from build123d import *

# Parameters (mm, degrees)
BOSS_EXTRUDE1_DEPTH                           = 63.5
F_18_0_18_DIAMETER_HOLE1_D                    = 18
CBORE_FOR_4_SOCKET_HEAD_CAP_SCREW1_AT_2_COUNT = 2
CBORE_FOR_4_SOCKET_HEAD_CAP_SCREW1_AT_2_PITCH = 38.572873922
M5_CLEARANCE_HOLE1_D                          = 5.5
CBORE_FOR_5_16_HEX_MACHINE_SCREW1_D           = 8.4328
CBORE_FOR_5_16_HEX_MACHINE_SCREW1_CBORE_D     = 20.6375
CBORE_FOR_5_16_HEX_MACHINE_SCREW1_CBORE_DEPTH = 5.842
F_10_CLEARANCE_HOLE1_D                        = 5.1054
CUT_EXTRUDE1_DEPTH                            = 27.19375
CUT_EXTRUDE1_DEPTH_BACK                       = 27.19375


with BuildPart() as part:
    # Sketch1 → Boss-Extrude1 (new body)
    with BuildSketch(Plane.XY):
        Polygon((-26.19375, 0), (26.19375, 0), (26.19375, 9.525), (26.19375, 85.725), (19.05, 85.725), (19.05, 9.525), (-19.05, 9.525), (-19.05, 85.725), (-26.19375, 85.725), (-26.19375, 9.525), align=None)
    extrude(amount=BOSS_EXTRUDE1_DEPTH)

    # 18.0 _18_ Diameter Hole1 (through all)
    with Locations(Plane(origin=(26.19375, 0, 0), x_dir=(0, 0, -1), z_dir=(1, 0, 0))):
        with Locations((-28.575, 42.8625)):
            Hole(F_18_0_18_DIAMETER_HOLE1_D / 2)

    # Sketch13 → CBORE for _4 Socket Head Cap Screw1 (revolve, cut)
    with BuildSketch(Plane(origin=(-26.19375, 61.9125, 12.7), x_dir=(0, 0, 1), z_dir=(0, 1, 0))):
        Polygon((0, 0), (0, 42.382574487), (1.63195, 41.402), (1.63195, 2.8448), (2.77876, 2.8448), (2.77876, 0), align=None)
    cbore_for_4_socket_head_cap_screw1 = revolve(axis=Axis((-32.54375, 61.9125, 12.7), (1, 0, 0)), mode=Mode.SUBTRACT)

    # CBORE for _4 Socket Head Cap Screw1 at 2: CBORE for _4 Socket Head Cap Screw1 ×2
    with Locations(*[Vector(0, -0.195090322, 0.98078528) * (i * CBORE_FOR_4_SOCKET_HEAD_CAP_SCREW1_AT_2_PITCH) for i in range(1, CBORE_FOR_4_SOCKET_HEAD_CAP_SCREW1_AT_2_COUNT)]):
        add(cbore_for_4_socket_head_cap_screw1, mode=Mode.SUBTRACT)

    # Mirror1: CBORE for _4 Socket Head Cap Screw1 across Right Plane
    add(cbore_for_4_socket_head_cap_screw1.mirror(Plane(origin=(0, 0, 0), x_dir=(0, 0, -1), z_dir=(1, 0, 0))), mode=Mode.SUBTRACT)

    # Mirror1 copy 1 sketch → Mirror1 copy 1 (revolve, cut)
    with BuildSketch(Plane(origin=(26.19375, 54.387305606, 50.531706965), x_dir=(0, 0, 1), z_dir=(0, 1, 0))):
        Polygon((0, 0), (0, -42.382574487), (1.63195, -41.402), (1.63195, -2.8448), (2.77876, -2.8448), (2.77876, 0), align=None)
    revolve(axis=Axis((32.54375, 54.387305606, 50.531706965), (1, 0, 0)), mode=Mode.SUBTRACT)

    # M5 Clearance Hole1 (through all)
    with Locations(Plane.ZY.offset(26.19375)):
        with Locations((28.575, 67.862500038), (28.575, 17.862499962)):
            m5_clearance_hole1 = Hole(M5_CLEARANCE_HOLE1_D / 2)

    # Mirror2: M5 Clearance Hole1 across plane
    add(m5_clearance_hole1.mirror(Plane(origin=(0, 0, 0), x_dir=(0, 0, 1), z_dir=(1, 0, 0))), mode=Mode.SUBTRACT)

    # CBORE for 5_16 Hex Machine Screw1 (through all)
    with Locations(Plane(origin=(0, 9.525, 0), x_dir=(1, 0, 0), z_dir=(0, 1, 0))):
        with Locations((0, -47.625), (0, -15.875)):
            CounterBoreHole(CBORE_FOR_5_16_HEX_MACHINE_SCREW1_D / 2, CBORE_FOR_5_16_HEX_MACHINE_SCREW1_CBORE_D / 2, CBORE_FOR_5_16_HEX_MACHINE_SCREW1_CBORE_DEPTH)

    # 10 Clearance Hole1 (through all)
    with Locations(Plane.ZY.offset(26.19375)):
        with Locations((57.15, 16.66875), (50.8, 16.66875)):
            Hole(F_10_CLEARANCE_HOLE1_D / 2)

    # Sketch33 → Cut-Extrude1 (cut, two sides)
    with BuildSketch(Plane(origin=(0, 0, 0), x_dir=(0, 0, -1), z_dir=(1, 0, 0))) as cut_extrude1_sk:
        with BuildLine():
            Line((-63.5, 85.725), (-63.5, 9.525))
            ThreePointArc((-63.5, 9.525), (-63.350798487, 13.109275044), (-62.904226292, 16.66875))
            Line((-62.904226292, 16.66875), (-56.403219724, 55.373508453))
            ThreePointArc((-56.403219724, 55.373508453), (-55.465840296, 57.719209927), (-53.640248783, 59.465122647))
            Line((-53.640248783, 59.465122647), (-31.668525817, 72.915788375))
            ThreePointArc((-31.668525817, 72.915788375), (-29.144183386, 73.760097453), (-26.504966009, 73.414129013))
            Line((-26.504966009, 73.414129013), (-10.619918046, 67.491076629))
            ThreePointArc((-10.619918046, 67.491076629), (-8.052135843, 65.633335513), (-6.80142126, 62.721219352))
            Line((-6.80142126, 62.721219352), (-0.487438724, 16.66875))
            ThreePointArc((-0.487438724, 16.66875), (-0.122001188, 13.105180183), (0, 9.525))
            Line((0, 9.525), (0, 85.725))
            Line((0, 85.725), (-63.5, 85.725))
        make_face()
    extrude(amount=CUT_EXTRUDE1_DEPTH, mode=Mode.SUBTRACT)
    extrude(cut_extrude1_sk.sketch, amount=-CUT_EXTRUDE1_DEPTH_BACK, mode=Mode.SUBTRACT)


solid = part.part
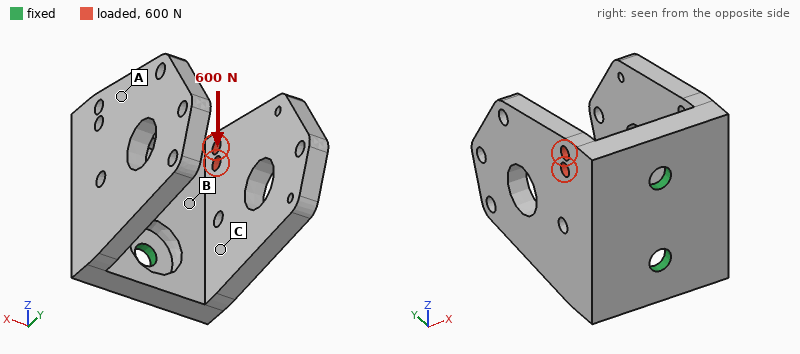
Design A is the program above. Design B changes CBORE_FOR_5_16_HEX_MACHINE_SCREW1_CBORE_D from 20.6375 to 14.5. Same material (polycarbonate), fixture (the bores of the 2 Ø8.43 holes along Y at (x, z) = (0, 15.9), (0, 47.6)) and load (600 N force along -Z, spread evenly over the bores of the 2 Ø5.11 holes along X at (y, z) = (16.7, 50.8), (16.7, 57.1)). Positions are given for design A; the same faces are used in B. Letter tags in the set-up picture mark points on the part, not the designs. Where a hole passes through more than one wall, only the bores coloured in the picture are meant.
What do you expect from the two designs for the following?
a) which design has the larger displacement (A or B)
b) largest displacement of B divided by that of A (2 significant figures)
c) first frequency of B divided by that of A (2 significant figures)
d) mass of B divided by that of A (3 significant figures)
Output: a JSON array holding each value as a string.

["A", "0.78", "1.1", "1.03"]
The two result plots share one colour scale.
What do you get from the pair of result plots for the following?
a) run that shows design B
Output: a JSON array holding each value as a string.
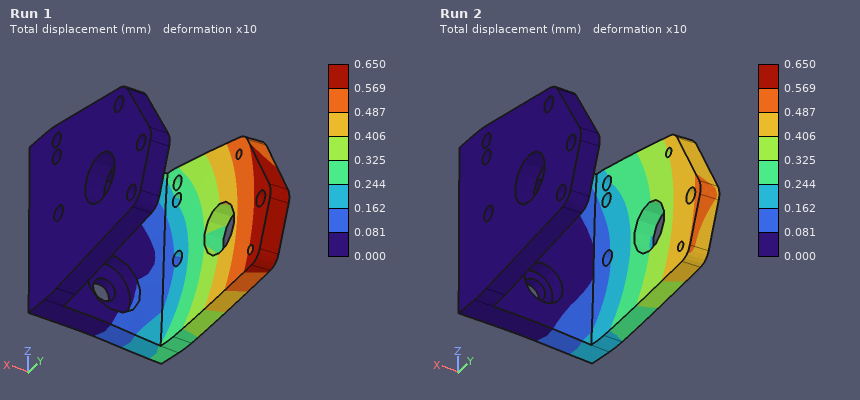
["Run 2"]
